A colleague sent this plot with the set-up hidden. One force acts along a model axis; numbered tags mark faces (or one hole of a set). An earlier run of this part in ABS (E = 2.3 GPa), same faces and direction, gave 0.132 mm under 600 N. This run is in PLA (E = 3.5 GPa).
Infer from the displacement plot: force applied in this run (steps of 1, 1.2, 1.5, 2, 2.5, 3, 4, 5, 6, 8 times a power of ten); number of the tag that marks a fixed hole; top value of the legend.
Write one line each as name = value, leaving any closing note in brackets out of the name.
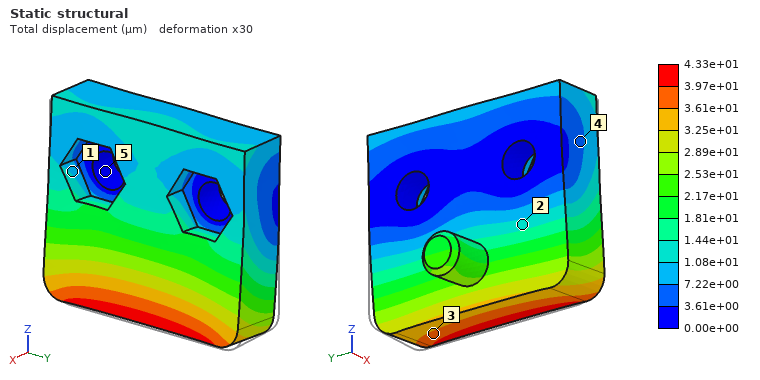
force applied in this run = 300 N
number of the tag that marks a fixed hole = 5
top value of the legend = 4.33e+01 µm
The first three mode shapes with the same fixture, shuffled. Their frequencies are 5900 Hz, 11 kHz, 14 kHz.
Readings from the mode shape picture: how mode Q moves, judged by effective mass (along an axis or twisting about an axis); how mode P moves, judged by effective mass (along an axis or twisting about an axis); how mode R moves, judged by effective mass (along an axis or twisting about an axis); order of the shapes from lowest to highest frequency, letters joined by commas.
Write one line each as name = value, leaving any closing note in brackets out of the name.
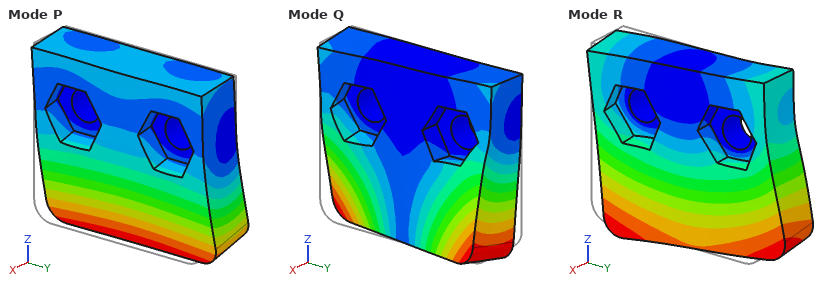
how mode Q moves, judged by effective mass = twisting about Z
how mode P moves, judged by effective mass = along X
how mode R moves, judged by effective mass = along Y
order of the shapes from lowest to highest frequency, letters joined by commas = P, Q, R
